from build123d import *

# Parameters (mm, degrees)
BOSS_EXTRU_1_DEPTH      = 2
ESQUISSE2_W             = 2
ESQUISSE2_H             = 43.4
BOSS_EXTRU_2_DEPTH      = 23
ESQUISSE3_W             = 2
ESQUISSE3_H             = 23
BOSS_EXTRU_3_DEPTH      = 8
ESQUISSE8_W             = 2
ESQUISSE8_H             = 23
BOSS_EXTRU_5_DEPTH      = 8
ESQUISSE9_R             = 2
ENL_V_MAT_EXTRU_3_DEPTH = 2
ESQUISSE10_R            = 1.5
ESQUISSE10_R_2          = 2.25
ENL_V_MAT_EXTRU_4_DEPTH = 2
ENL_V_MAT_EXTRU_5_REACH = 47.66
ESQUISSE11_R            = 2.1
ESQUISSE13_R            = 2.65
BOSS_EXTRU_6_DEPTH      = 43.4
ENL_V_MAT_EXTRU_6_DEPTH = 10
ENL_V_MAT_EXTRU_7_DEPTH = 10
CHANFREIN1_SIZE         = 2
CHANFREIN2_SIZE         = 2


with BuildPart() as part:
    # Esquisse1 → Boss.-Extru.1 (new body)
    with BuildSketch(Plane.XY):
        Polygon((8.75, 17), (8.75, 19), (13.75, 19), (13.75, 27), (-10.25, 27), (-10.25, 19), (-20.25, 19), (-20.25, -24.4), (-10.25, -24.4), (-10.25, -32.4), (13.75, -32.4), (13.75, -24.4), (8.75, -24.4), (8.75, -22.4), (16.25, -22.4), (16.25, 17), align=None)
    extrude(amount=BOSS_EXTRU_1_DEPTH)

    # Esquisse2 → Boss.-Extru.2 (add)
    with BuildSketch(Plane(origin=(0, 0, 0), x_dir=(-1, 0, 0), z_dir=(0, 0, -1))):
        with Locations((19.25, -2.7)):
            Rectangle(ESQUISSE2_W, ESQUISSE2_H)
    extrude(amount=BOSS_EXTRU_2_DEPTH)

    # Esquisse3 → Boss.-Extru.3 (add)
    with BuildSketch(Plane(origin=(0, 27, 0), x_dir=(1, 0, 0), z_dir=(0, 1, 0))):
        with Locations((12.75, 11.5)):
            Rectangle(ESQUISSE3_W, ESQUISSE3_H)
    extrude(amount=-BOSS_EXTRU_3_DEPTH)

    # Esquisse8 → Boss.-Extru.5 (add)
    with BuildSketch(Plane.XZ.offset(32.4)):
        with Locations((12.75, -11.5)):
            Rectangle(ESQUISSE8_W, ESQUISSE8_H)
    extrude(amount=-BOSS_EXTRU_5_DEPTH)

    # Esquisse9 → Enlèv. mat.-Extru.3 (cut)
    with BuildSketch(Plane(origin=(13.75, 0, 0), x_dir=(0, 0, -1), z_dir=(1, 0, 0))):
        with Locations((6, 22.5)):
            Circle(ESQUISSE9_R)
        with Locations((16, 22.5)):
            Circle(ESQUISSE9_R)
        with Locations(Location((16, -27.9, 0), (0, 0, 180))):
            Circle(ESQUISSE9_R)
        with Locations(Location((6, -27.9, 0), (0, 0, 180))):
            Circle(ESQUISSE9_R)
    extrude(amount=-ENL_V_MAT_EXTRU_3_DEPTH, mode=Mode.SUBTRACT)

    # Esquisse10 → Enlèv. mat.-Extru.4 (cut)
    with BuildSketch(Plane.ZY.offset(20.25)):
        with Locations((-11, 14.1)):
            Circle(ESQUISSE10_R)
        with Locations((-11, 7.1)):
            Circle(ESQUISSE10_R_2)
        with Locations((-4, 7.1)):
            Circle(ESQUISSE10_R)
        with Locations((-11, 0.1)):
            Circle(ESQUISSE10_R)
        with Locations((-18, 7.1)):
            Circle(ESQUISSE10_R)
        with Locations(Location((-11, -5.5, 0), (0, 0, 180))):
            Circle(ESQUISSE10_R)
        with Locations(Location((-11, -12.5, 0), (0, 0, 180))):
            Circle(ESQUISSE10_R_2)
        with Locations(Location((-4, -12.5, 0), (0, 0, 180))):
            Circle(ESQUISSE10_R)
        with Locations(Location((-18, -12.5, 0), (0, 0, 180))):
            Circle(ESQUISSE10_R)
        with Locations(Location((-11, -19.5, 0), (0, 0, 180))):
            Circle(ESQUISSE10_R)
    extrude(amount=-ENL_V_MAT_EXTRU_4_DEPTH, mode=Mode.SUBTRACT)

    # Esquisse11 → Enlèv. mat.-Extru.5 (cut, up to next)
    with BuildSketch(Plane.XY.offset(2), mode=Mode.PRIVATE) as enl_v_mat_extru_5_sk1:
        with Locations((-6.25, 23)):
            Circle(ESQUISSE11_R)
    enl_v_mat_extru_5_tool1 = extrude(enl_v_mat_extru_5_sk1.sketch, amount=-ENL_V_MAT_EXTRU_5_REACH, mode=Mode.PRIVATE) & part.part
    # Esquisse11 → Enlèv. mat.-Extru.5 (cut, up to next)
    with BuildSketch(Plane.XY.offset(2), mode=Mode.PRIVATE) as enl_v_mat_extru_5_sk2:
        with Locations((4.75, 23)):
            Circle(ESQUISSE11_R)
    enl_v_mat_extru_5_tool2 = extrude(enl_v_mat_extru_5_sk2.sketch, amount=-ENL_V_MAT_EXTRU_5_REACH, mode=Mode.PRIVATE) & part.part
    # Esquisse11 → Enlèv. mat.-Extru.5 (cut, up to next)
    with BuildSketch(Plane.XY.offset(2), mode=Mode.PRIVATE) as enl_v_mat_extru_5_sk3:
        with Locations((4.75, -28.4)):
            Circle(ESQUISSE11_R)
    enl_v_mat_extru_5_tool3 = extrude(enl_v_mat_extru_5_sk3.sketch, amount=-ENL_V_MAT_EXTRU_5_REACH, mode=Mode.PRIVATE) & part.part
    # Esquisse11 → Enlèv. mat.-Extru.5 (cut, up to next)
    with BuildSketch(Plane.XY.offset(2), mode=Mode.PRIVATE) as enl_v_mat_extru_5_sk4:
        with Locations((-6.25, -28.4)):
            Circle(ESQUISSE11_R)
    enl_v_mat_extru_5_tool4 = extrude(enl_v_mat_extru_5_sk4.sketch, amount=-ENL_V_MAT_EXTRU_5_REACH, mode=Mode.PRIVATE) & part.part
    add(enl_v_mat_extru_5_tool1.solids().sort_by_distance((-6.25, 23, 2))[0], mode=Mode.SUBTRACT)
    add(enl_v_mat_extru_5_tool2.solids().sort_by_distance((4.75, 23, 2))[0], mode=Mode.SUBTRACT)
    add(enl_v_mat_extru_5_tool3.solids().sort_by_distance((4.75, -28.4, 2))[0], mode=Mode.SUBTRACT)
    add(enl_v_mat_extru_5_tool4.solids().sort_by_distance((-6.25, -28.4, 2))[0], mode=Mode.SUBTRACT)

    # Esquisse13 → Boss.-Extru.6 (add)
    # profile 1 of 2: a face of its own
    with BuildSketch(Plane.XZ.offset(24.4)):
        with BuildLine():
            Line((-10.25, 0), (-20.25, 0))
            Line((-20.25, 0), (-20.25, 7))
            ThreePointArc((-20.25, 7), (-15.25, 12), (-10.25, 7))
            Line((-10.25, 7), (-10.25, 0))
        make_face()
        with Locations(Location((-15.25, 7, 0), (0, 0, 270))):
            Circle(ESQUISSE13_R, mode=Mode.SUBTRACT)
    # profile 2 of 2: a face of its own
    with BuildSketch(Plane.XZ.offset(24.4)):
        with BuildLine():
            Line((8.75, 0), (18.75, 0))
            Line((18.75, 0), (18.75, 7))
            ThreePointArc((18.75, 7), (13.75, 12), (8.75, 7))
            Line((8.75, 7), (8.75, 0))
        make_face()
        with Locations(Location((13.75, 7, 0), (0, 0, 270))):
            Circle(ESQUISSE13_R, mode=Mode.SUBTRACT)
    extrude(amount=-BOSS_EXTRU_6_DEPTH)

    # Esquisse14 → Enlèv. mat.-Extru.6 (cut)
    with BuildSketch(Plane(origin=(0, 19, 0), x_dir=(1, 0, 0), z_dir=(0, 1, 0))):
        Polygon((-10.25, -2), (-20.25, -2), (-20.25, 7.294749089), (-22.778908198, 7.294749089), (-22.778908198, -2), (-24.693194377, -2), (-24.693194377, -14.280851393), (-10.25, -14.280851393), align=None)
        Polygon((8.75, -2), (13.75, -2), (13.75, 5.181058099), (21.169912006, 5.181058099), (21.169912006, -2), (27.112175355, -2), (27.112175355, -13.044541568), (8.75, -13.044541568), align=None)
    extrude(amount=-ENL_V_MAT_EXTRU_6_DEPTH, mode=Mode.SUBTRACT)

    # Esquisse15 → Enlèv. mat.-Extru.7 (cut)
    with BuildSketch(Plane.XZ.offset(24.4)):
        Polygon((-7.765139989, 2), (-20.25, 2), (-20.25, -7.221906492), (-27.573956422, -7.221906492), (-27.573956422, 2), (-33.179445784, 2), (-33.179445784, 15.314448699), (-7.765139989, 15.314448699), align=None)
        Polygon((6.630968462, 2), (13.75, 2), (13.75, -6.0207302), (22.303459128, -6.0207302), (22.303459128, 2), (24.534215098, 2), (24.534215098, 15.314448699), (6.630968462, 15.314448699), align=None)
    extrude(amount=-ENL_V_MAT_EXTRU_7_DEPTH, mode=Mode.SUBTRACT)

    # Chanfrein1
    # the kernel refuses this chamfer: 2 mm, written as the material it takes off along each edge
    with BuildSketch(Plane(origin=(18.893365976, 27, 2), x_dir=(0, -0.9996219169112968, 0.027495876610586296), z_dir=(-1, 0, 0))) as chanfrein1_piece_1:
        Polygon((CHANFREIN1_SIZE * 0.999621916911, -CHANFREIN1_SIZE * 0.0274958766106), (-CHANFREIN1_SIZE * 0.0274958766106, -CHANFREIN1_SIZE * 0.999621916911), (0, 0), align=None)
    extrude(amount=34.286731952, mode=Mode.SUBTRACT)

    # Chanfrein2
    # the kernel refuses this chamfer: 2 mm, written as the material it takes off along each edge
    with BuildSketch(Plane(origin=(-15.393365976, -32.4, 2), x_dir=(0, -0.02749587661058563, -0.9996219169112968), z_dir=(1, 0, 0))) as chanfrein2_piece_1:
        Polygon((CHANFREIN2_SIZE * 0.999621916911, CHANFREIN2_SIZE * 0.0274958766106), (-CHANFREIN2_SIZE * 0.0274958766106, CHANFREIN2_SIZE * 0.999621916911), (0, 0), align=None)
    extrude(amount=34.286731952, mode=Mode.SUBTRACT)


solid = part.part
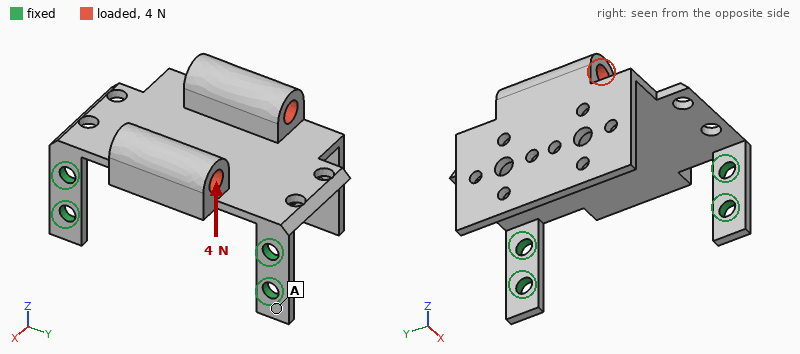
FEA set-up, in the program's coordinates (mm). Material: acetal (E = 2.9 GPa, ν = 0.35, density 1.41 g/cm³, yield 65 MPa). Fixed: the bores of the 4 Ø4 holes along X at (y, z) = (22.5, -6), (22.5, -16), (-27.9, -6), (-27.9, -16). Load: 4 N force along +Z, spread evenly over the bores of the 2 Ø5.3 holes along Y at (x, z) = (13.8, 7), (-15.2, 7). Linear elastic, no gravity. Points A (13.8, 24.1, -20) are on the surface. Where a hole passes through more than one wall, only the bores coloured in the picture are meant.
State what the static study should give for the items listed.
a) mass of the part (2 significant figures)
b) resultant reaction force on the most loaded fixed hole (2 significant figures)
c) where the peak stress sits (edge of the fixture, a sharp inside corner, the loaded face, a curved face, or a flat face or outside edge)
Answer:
13 g
2.1 N
a curved face
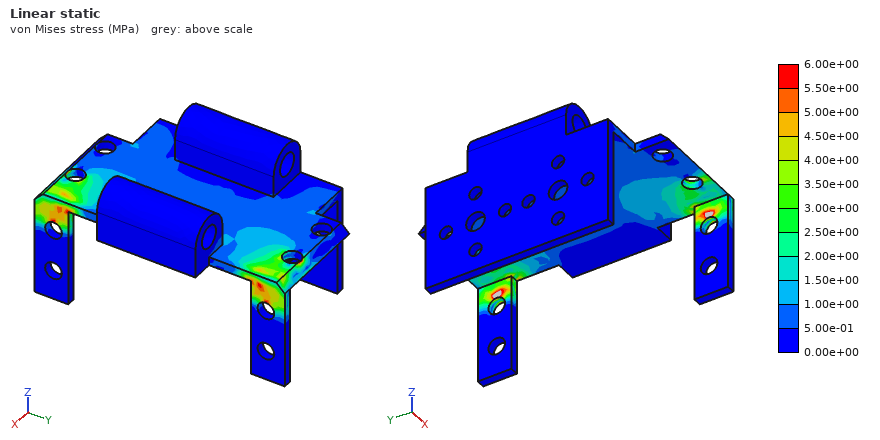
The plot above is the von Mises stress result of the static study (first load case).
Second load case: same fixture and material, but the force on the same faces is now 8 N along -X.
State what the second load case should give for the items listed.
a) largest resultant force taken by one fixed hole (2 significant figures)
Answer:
4.6 N
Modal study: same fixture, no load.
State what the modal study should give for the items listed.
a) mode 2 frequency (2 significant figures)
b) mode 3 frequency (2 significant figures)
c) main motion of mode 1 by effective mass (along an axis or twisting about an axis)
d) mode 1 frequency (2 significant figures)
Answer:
450 Hz
540 Hz
along Z
100 Hz
